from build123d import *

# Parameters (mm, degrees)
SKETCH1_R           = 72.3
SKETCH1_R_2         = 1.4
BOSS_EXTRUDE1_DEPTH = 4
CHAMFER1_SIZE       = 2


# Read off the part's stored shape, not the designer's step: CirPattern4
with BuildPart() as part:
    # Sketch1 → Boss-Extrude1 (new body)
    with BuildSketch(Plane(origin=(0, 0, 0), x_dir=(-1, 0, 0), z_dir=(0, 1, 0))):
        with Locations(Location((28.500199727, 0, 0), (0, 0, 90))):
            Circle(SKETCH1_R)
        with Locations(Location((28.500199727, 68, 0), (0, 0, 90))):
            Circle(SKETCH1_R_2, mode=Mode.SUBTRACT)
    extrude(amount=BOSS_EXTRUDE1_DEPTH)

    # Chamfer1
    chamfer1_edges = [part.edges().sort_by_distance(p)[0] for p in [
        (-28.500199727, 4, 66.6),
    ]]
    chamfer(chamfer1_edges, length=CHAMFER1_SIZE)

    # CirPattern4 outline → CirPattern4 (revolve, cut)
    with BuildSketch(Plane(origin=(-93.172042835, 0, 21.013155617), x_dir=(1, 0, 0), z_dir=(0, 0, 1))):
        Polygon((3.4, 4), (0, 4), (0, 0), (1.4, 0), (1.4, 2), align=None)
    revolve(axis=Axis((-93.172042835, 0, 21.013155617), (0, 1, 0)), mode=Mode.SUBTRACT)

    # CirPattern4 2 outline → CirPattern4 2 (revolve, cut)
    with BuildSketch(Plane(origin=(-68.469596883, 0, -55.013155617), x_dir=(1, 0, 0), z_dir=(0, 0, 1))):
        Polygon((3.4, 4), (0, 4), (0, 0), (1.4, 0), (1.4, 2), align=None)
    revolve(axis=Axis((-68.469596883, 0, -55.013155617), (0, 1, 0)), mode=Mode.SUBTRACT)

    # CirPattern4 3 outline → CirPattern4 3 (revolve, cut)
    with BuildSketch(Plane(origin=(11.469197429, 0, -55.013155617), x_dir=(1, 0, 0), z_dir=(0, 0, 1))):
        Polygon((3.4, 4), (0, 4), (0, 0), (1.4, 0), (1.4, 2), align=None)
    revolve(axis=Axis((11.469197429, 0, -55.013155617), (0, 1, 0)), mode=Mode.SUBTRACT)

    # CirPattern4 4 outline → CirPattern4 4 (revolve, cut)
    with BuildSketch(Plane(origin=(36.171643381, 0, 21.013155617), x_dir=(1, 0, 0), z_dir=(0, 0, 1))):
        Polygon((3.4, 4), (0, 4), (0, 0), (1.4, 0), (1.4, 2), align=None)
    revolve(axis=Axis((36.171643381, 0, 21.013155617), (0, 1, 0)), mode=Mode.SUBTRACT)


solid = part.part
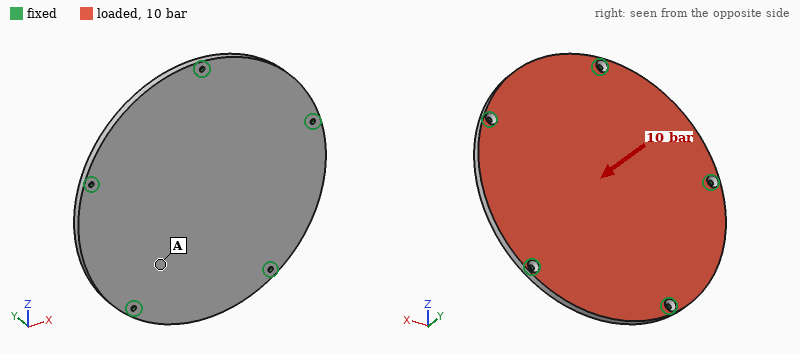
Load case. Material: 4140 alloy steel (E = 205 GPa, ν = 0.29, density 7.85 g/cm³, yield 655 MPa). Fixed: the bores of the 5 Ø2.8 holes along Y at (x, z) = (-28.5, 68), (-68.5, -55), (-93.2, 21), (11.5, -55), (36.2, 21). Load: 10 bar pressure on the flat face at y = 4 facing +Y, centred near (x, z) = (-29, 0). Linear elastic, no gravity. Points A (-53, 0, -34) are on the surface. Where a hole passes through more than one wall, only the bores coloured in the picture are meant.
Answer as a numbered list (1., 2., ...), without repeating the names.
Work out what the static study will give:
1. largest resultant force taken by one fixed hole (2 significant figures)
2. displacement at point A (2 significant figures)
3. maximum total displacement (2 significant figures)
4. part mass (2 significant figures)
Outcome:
1. 5.4 kN
2. 0.37 mm
3. 0.69 mm
4. 510 g
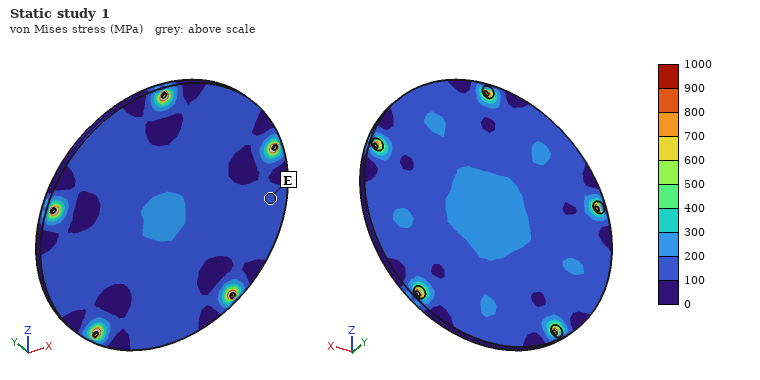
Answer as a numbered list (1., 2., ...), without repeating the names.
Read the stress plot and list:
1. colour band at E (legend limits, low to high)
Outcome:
1. 100 to 200 MPa
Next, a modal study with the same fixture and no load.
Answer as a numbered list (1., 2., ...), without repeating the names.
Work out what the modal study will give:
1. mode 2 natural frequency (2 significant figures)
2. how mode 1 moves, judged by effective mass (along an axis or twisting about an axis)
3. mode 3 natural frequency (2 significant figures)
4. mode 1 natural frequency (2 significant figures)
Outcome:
1. 2400 Hz
2. along Y
3. 2400 Hz
4. 1300 Hz
